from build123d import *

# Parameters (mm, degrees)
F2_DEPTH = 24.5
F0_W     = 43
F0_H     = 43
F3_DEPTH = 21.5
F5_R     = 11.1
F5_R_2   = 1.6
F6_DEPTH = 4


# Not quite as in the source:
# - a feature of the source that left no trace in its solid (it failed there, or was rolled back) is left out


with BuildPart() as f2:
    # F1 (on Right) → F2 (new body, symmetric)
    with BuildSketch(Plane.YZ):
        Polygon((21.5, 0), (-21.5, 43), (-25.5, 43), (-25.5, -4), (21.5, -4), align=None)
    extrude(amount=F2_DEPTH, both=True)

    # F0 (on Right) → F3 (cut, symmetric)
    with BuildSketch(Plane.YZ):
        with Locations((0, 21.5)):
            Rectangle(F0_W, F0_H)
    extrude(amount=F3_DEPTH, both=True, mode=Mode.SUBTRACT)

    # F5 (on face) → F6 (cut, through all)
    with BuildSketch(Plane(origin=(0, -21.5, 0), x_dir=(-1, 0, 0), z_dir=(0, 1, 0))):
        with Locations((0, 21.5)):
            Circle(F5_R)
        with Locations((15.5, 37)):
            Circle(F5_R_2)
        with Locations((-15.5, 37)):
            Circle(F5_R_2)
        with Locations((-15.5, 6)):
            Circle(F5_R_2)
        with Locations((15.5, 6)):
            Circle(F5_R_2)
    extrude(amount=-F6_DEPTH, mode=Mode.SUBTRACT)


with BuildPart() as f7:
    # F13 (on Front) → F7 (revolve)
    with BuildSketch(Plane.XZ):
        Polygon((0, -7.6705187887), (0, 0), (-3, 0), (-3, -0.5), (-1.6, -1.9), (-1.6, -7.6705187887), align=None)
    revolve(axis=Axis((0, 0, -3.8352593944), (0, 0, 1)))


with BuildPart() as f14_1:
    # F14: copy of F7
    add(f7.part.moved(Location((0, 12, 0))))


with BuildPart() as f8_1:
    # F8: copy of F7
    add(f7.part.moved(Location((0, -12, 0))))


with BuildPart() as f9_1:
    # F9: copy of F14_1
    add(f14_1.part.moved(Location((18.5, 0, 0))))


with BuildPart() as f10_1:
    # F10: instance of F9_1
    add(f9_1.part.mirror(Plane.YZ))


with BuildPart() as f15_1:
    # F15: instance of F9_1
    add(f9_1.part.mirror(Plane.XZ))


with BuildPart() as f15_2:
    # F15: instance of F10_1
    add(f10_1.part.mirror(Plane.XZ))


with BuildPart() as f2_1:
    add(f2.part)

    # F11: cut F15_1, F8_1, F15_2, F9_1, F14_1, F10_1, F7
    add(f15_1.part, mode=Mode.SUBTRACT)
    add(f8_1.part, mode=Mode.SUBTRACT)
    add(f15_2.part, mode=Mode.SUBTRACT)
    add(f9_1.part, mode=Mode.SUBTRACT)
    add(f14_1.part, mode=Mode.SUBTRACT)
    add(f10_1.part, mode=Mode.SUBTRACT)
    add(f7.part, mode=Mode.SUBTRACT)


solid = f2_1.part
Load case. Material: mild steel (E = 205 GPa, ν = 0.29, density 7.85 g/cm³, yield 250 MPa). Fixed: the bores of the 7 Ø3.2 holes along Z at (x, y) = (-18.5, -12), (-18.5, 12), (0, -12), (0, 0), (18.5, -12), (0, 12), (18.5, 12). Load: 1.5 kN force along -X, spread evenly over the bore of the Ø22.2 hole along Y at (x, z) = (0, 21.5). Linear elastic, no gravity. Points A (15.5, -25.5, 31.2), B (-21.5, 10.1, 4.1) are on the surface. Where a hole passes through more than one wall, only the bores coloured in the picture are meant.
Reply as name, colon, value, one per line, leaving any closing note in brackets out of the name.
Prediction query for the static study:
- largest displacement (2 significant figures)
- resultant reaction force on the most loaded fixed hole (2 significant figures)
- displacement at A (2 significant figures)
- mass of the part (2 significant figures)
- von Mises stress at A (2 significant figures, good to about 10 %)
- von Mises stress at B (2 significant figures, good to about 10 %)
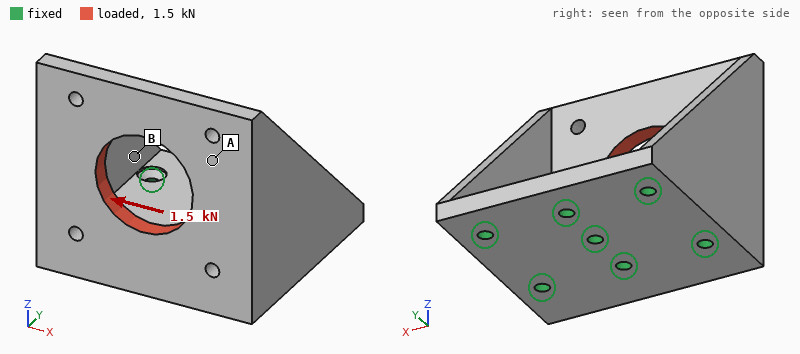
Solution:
largest displacement: 29 µm
resultant reaction force on the most loaded fixed hole: 1.3 kN
displacement at A: 20 µm
mass of the part: 170 g
von Mises stress at A: 9.0 MPa
von Mises stress at B: 22 MPa
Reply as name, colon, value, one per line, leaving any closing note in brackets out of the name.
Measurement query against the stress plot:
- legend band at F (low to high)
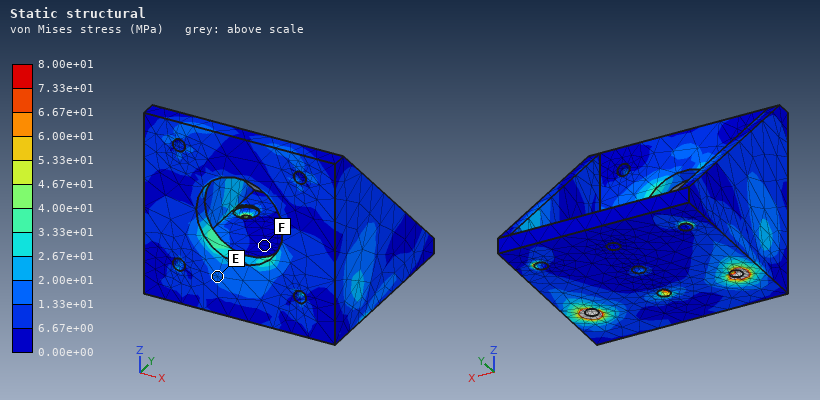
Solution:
legend band at F: 0.00e+00 to 6.67e+00 MPa
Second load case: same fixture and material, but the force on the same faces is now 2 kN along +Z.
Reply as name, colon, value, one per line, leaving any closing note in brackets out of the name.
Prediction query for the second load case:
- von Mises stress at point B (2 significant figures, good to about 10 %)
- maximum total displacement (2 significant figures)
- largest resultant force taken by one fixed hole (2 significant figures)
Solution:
von Mises stress at point B: 19 MPa
maximum total displacement: 20 µm
largest resultant force taken by one fixed hole: 1.3 kN
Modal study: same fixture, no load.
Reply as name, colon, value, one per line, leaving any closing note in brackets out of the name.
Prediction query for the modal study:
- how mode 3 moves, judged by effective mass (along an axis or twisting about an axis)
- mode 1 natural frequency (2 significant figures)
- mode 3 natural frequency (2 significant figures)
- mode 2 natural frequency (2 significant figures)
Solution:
how mode 3 moves, judged by effective mass: along Z
mode 1 natural frequency: 4400 Hz
mode 3 natural frequency: 7400 Hz
mode 2 natural frequency: 4400 Hz
